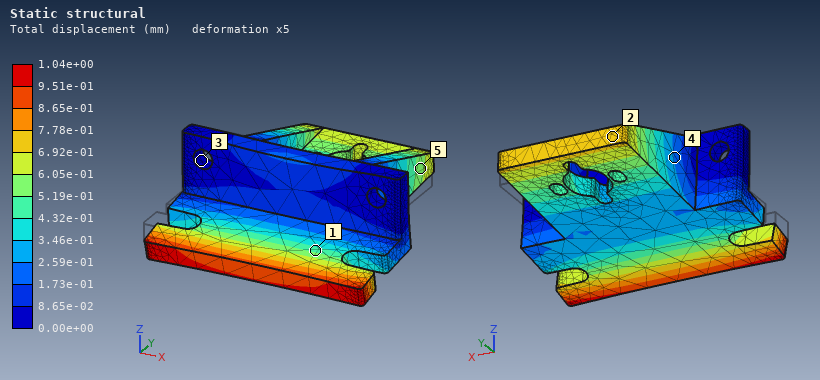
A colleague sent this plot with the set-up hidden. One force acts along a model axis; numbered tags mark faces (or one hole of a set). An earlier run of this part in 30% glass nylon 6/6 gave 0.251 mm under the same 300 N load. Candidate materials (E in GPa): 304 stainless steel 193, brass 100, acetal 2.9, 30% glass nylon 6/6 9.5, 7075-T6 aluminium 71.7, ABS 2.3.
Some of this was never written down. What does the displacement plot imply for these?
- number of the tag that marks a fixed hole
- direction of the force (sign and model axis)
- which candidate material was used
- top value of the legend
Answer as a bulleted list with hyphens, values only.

- 3
- -Z
- ABS
- 1.04e+00 mm
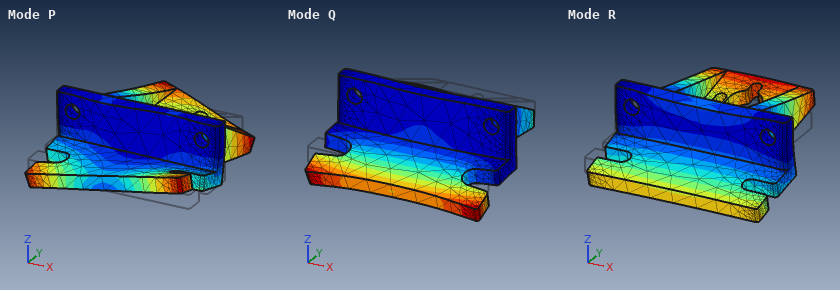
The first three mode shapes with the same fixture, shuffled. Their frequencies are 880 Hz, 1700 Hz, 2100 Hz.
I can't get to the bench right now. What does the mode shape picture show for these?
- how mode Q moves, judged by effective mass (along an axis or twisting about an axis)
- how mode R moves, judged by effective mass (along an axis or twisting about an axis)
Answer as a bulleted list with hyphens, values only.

- along Z
- along Y
